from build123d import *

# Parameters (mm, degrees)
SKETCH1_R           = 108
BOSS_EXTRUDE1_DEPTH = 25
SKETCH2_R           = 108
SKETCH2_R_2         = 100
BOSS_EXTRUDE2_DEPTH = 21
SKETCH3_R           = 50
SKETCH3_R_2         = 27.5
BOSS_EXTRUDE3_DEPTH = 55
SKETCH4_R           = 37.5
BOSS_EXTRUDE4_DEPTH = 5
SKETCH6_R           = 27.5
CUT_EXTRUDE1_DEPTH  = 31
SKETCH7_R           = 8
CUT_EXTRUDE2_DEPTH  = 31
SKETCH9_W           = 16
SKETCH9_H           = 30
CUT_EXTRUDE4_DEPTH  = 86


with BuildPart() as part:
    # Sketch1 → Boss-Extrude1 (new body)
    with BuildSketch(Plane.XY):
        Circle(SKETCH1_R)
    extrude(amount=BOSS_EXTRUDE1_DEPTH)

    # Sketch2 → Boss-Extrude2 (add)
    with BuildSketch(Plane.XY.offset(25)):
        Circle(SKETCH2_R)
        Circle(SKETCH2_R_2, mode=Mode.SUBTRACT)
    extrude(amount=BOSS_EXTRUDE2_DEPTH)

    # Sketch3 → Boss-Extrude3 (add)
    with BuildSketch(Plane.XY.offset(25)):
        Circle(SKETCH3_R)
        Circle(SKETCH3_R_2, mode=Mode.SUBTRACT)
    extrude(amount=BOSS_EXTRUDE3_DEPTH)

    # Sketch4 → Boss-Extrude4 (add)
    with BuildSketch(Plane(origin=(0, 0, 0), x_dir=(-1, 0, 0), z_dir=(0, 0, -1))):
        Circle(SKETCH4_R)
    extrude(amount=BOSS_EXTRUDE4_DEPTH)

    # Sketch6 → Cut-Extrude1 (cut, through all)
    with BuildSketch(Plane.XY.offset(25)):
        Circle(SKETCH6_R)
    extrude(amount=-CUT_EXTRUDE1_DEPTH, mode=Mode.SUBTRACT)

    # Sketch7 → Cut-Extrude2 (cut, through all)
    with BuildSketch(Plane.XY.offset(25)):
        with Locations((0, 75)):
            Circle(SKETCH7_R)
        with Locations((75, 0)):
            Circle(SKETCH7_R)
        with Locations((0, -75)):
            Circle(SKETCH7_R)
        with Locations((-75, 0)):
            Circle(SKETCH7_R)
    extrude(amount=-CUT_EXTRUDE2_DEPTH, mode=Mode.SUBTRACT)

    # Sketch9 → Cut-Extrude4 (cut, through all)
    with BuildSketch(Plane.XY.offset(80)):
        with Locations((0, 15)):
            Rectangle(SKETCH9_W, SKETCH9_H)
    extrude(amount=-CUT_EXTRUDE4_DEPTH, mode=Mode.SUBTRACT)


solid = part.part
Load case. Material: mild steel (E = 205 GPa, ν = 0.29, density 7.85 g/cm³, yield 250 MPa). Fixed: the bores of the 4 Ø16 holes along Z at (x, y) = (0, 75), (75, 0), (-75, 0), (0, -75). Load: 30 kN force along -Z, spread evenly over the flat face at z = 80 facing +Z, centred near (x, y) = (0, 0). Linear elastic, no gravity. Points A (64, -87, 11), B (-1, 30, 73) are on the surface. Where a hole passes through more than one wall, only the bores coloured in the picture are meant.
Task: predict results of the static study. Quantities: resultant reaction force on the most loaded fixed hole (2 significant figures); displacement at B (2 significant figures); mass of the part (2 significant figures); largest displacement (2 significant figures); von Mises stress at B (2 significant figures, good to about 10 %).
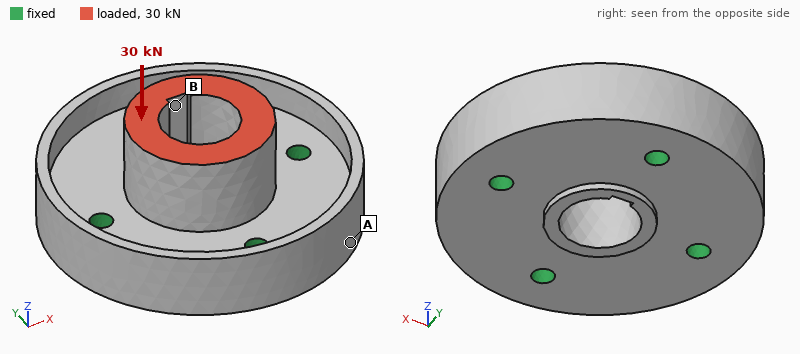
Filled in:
7.8 kN
5.1 µm
9.8 kg
5.6 µm
5.6 MPa
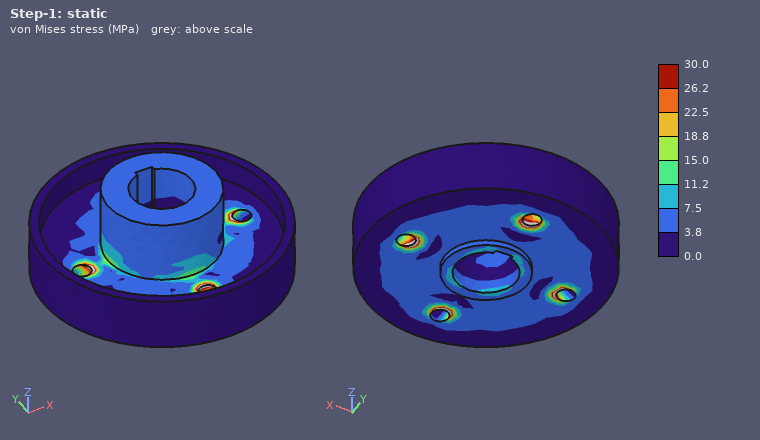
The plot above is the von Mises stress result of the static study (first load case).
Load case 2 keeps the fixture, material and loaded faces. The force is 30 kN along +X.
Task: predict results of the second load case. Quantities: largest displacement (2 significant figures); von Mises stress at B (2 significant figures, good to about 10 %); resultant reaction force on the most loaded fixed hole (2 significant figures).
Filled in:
22 µm
30 MPa
17 kN
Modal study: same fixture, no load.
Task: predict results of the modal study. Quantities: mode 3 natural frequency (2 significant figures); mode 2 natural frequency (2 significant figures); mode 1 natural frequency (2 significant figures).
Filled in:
5300 Hz
5300 Hz
4900 Hz
